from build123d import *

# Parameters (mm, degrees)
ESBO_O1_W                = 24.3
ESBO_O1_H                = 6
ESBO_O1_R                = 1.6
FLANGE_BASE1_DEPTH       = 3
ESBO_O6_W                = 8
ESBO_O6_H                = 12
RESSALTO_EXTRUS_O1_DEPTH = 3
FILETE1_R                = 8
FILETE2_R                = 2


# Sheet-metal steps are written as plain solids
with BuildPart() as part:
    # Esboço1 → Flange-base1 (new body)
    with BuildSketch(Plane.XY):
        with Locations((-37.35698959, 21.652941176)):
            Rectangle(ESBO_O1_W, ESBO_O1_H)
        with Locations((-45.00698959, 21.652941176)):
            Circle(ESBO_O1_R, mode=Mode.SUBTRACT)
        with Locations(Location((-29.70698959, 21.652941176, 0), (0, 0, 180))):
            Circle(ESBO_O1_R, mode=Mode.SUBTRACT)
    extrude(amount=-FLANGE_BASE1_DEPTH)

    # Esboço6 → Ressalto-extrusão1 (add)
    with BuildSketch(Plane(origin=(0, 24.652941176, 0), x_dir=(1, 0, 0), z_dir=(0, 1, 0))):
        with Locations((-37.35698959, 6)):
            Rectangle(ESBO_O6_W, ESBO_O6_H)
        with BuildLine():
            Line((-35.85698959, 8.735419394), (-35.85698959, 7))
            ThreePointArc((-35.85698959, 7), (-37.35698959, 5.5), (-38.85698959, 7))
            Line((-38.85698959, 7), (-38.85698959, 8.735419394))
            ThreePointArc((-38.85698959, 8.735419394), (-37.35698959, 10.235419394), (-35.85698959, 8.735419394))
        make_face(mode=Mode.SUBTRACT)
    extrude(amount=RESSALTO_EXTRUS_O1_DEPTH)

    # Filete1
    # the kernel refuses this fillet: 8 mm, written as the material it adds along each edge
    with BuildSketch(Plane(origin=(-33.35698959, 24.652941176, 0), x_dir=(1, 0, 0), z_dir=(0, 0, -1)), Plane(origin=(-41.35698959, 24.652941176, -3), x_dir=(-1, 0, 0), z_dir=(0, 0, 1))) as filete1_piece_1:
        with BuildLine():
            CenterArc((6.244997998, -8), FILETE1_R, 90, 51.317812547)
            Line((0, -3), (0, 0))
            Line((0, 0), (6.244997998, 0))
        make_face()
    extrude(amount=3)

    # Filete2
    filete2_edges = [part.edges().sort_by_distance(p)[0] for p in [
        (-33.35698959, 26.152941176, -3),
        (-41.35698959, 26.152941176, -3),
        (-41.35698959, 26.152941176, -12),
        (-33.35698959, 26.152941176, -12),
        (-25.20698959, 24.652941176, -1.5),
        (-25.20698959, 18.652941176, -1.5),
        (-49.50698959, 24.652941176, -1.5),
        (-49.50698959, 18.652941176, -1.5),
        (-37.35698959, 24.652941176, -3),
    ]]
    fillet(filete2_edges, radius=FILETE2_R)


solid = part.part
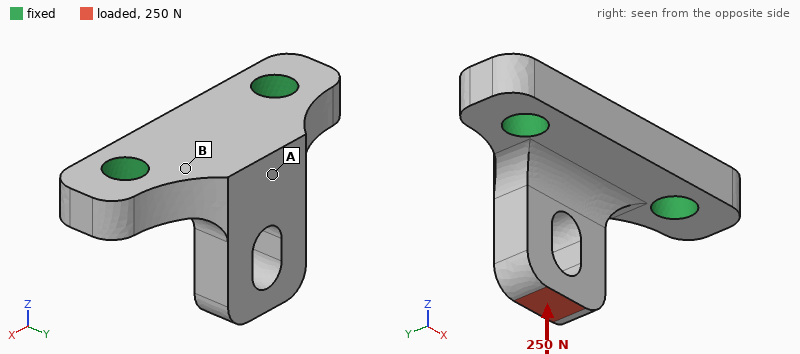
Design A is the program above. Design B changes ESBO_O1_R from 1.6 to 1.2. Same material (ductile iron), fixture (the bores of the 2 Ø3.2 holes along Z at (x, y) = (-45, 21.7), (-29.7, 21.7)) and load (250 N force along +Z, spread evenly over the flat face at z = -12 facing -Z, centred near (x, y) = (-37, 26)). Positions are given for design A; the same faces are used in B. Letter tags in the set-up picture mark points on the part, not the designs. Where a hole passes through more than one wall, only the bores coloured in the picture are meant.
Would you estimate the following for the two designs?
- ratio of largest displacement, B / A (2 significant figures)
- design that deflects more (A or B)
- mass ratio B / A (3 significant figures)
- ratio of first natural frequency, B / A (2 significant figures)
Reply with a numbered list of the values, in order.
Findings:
1. 1.2
2. B
3. 1.03
4. 0.95
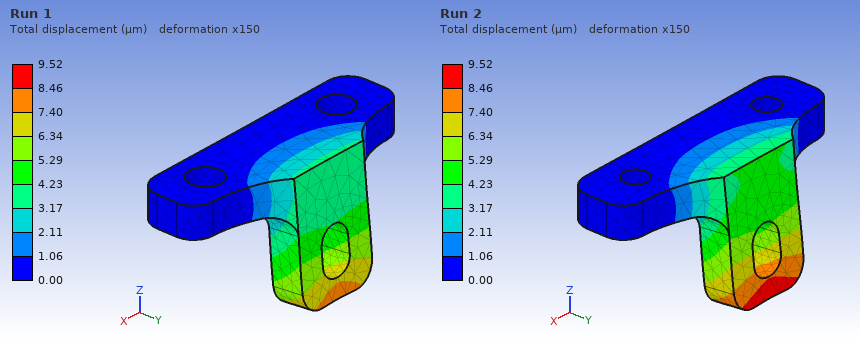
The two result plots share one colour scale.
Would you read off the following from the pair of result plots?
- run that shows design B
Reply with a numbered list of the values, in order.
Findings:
1. Run 2
